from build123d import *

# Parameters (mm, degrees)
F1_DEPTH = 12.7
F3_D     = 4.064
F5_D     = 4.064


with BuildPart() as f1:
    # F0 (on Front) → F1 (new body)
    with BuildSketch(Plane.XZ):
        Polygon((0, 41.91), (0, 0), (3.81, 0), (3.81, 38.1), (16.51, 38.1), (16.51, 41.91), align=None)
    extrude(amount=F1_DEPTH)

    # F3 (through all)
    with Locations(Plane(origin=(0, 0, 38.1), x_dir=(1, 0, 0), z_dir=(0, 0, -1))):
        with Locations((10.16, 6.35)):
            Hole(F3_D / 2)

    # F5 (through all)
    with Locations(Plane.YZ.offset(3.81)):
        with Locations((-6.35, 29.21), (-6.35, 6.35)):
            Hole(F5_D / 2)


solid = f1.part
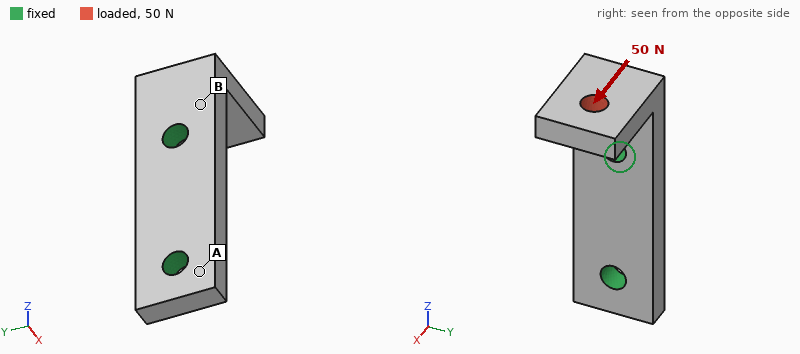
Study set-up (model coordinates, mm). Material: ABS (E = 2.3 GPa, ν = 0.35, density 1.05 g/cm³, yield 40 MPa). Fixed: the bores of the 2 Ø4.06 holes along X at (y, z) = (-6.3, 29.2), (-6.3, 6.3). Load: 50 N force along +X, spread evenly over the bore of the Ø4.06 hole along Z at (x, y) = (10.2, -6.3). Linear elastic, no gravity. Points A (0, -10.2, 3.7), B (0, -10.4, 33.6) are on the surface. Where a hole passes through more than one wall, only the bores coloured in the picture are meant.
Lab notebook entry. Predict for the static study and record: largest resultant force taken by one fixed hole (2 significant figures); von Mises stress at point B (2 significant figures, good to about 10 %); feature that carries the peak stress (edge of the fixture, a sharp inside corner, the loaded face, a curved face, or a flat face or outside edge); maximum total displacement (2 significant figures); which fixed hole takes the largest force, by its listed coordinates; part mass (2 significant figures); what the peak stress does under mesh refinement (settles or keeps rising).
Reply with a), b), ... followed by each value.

a) 52 N
b) 8.7 MPa
c) edge of the fixture
d) 0.32 mm
e) (-6.3, 29.2)
f) 2.6 g
g) keeps rising
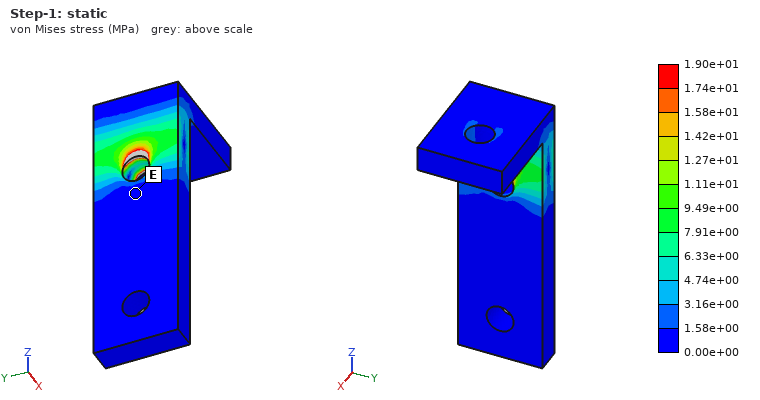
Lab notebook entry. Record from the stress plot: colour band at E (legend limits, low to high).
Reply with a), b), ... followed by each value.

a) 0.00e+00 to 1.58e+00 MPa
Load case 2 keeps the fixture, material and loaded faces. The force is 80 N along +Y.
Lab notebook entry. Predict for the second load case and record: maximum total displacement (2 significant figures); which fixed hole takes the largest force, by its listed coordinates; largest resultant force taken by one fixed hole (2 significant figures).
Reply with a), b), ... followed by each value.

a) 0.56 mm
b) (-6.3, 29.2)
c) 97 N
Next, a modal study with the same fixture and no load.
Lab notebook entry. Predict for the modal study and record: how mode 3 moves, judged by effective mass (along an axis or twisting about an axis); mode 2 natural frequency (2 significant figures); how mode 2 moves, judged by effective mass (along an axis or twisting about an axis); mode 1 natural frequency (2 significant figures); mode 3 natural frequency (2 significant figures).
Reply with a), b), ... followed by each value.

a) along X
b) 2800 Hz
c) along Y
d) 2100 Hz
e) 5600 Hz
